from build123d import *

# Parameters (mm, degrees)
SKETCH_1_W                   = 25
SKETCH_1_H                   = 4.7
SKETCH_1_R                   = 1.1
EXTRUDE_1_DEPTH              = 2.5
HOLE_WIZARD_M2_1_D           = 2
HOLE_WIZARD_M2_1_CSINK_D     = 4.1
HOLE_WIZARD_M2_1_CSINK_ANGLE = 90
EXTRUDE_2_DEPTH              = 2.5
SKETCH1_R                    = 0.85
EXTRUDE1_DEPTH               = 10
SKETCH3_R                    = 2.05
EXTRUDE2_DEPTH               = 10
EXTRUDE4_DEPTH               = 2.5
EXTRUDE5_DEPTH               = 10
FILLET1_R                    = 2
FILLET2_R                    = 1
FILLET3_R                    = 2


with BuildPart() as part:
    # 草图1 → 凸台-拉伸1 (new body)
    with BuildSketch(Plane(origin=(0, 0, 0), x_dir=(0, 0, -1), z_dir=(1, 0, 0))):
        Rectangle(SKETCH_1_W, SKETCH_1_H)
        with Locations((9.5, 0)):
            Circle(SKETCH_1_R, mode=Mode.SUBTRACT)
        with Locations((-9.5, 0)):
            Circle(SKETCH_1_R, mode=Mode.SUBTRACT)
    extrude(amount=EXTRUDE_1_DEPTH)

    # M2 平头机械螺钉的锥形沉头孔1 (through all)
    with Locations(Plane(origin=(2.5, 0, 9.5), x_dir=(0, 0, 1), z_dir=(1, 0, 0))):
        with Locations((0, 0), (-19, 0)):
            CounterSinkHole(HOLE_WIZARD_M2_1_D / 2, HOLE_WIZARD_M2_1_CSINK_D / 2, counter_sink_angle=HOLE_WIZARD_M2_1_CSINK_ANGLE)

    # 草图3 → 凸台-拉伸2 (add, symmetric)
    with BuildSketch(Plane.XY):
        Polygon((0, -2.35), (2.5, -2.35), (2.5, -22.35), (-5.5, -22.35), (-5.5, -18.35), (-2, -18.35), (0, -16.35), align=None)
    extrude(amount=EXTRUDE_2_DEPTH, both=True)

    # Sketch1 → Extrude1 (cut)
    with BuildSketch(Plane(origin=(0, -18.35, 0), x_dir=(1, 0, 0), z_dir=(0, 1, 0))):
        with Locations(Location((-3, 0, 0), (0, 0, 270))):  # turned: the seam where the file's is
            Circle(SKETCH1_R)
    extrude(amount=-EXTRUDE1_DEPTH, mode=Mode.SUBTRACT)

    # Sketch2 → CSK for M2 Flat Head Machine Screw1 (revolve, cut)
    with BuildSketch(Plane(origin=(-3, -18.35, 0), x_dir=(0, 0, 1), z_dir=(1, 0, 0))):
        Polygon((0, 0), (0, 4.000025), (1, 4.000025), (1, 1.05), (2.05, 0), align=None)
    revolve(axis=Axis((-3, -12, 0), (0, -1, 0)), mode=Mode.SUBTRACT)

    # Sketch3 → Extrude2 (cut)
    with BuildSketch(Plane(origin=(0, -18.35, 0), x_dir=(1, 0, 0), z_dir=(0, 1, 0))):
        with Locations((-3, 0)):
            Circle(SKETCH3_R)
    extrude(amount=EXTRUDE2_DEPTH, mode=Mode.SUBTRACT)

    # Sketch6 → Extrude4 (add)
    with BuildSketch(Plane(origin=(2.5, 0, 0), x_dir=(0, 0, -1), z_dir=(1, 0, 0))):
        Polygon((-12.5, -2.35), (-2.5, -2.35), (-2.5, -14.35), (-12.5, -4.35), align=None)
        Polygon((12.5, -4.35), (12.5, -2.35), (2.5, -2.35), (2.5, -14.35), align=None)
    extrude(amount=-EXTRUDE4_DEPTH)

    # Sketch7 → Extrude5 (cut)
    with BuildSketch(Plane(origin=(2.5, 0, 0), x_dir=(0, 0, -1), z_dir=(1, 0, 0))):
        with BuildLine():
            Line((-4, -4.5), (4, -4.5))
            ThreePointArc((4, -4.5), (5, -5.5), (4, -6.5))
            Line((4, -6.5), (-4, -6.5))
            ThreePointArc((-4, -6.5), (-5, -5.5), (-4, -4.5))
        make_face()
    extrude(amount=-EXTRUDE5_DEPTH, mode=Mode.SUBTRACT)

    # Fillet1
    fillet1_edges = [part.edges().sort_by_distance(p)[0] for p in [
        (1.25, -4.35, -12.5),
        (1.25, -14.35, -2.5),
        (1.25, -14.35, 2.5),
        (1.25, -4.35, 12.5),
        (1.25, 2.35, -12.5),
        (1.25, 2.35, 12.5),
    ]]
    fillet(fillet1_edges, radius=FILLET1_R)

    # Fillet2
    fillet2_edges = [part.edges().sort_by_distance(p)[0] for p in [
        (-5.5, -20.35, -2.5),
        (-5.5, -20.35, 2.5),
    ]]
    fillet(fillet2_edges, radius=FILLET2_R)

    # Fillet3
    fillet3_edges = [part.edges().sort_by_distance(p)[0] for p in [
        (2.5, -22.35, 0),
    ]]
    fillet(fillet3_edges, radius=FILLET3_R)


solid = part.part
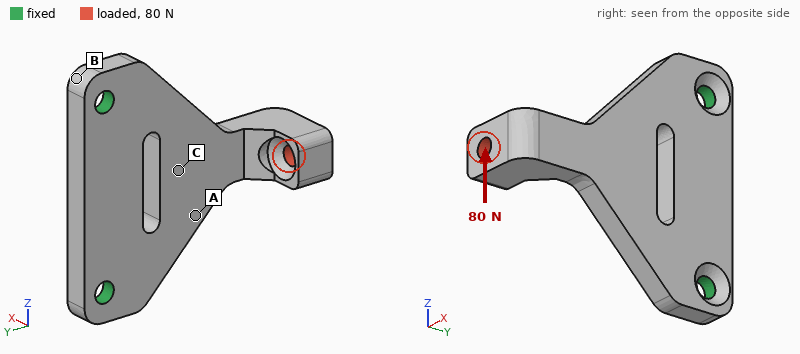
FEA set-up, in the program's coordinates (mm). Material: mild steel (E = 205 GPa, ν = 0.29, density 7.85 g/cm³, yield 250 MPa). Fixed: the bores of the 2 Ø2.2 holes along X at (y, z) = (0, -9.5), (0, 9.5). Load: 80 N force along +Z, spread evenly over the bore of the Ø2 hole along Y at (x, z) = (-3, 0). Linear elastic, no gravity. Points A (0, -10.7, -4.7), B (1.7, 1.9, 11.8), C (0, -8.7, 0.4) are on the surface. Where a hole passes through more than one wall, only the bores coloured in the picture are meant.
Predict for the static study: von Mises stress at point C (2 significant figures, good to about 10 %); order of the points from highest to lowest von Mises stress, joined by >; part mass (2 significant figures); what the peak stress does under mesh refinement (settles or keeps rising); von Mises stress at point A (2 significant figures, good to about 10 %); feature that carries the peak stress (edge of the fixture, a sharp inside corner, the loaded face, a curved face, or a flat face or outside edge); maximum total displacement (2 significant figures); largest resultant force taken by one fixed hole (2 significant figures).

16 MPa
A > C > B
7.1 g
keeps rising
32 MPa
edge of the fixture
17 µm
95 N
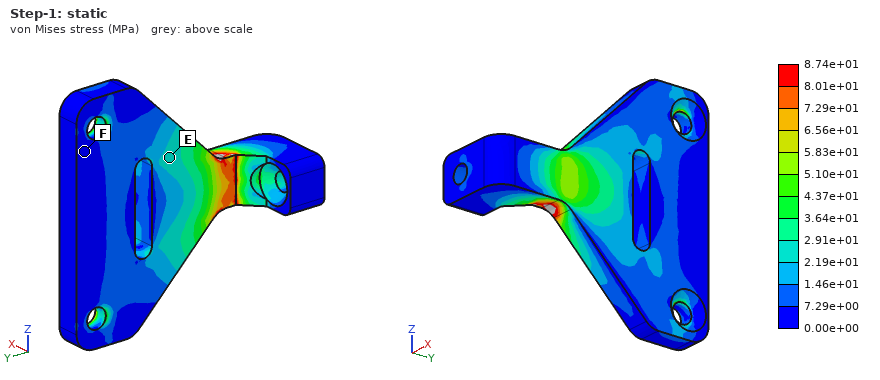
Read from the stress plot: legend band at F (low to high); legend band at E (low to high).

0.00e+00 to 7.29e+00 MPa
2.19e+01 to 2.91e+01 MPa
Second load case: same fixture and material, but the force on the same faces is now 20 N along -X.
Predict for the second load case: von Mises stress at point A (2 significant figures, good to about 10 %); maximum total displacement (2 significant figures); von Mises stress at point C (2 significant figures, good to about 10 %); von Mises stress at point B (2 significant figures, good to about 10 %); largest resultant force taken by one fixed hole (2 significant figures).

21 MPa
32 µm
11 MPa
6.8 MPa
10 N
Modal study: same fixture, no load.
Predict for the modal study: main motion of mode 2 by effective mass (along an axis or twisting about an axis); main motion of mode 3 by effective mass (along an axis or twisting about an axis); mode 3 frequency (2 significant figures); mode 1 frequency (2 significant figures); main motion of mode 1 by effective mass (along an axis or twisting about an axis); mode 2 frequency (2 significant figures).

along Z
along X
15 kHz
3600 Hz
along X
14 kHz
